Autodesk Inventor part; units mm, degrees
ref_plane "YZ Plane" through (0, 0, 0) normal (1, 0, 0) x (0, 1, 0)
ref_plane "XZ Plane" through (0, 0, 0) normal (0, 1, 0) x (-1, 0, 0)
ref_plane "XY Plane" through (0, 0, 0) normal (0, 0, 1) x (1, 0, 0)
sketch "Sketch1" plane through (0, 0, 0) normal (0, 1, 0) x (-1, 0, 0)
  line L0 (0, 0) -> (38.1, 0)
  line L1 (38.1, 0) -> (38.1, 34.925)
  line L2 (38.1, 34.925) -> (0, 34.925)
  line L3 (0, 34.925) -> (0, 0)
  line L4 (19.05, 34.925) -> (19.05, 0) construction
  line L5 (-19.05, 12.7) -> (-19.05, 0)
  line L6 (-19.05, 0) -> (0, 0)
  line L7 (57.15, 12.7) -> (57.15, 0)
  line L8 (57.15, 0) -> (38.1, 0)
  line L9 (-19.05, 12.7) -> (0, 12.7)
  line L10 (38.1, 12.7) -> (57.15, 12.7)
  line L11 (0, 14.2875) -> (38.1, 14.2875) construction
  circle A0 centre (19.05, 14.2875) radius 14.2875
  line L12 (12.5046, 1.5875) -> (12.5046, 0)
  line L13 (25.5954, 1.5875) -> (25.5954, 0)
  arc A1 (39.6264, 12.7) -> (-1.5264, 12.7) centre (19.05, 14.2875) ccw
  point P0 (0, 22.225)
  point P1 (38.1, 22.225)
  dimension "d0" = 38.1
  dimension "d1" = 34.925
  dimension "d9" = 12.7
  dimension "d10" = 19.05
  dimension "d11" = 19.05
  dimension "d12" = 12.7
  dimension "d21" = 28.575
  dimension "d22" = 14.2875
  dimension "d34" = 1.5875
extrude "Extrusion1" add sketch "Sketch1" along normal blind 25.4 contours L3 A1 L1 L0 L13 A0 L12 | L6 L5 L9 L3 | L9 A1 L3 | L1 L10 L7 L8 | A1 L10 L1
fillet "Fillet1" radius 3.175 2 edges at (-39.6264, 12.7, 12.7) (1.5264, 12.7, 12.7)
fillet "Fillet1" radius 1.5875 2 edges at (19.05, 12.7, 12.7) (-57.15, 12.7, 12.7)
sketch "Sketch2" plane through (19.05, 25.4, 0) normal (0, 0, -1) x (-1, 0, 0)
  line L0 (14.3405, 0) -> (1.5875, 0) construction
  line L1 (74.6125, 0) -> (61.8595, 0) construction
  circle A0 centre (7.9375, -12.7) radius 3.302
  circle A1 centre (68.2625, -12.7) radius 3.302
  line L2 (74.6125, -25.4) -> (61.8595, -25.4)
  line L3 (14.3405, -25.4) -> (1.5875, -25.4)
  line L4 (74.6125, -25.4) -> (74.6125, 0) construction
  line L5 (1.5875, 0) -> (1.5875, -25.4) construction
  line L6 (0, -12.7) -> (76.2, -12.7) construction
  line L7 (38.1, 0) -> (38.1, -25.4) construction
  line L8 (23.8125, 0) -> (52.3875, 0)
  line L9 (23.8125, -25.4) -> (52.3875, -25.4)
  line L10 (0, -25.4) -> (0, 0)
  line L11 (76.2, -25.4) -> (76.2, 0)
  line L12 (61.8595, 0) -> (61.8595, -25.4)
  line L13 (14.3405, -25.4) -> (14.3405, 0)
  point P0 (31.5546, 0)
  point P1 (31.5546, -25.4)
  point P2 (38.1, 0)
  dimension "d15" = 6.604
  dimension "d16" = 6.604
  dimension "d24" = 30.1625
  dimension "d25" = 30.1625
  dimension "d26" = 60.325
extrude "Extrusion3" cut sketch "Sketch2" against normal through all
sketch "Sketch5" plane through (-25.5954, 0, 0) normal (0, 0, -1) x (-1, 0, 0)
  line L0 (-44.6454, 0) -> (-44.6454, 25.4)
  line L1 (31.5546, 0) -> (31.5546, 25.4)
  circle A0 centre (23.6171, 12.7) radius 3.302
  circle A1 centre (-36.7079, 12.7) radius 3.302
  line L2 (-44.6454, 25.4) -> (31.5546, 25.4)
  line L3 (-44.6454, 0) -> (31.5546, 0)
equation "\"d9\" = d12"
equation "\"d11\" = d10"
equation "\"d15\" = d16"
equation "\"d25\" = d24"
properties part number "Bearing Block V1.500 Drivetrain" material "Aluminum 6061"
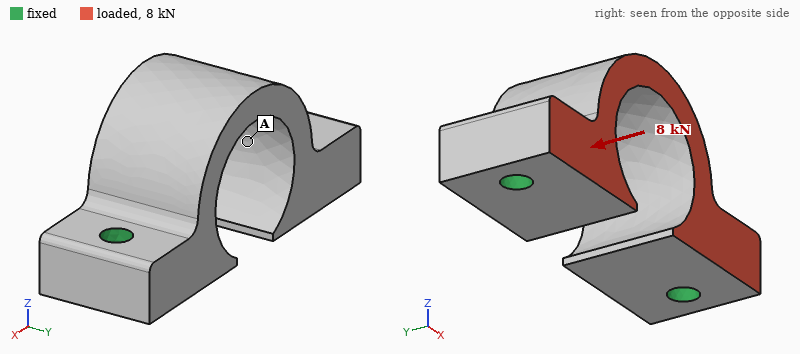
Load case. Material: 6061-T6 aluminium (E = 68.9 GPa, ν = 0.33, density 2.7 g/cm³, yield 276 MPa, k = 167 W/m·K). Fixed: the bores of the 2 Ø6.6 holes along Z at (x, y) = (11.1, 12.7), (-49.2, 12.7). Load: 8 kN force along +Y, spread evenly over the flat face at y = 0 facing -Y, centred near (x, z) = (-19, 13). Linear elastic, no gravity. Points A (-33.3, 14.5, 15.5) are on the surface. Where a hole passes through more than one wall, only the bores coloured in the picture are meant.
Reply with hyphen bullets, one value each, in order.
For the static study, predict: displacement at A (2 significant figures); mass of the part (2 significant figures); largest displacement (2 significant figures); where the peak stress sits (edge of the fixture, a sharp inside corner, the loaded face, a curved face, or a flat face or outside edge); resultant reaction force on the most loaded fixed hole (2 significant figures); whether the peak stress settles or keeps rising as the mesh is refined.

- 24 µm
- 70 g
- 61 µm
- edge of the fixture
- 4.0 kN
- keeps rising
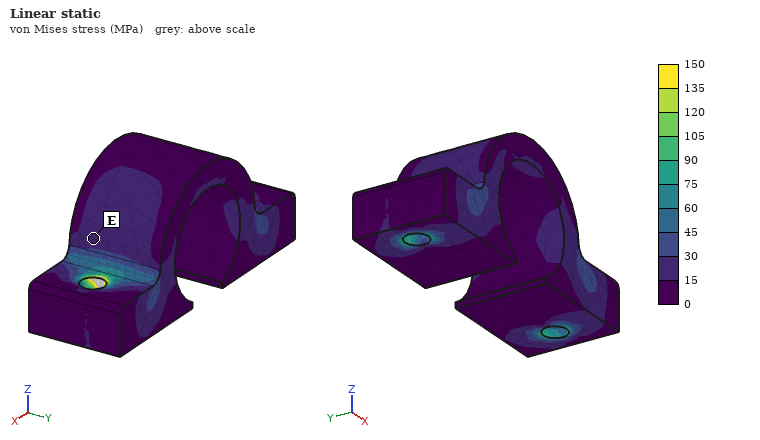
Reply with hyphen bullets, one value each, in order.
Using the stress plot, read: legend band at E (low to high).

- 15 to 30 MPa
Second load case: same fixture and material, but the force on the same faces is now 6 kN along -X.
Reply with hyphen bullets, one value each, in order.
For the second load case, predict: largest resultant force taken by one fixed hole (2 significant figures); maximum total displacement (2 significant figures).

- 3.1 kN
- 31 µm
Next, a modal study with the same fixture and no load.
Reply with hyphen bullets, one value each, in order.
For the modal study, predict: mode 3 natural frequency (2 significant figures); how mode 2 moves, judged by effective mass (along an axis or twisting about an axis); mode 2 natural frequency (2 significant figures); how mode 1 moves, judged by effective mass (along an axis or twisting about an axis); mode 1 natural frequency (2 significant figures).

- 16 kHz
- along X
- 12 kHz
- along Y
- 8300 Hz
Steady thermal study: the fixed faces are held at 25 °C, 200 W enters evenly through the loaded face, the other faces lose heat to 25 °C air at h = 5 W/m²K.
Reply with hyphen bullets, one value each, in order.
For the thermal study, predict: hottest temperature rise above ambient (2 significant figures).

- 47 K
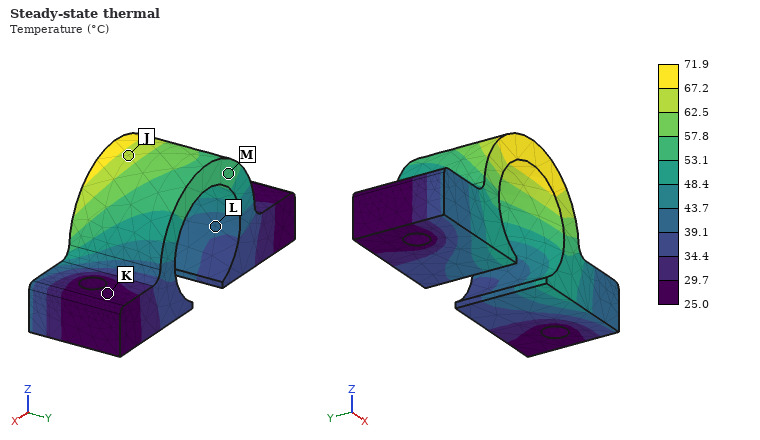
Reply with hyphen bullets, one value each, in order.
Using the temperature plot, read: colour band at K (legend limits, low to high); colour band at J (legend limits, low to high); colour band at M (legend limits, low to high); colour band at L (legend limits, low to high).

- 25.0 to 29.7 °C
- 62.5 to 67.2 °C
- 53.1 to 57.8 °C
- 39.1 to 43.7 °C
